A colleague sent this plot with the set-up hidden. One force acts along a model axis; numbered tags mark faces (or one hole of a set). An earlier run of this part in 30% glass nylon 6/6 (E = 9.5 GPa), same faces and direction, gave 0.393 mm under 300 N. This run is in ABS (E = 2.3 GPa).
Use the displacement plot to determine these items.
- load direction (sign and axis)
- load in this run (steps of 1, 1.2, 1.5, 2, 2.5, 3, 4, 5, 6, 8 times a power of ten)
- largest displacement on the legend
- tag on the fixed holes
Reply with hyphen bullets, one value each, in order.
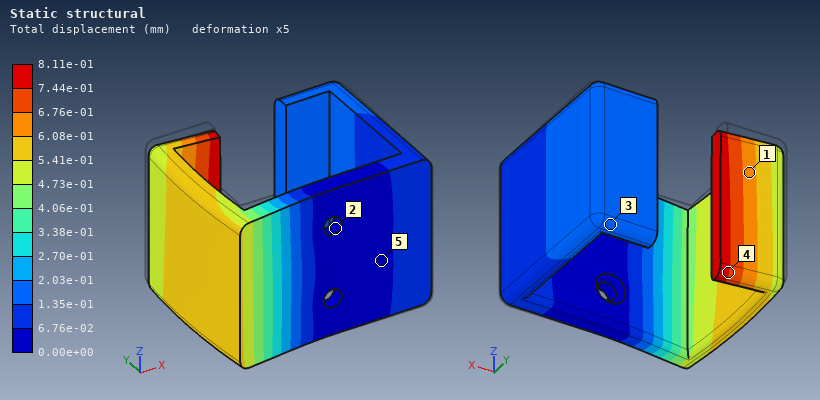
- -Y
- 150 N
- 8.11e-01 mm
- 2
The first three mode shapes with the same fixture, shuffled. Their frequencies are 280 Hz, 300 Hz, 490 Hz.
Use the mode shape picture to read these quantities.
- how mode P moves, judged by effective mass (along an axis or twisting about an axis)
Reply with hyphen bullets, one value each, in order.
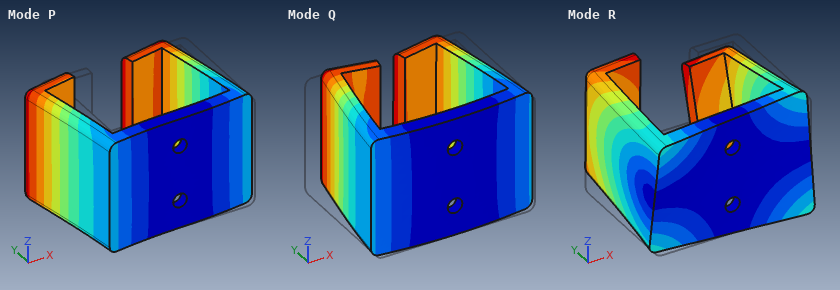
- along X
